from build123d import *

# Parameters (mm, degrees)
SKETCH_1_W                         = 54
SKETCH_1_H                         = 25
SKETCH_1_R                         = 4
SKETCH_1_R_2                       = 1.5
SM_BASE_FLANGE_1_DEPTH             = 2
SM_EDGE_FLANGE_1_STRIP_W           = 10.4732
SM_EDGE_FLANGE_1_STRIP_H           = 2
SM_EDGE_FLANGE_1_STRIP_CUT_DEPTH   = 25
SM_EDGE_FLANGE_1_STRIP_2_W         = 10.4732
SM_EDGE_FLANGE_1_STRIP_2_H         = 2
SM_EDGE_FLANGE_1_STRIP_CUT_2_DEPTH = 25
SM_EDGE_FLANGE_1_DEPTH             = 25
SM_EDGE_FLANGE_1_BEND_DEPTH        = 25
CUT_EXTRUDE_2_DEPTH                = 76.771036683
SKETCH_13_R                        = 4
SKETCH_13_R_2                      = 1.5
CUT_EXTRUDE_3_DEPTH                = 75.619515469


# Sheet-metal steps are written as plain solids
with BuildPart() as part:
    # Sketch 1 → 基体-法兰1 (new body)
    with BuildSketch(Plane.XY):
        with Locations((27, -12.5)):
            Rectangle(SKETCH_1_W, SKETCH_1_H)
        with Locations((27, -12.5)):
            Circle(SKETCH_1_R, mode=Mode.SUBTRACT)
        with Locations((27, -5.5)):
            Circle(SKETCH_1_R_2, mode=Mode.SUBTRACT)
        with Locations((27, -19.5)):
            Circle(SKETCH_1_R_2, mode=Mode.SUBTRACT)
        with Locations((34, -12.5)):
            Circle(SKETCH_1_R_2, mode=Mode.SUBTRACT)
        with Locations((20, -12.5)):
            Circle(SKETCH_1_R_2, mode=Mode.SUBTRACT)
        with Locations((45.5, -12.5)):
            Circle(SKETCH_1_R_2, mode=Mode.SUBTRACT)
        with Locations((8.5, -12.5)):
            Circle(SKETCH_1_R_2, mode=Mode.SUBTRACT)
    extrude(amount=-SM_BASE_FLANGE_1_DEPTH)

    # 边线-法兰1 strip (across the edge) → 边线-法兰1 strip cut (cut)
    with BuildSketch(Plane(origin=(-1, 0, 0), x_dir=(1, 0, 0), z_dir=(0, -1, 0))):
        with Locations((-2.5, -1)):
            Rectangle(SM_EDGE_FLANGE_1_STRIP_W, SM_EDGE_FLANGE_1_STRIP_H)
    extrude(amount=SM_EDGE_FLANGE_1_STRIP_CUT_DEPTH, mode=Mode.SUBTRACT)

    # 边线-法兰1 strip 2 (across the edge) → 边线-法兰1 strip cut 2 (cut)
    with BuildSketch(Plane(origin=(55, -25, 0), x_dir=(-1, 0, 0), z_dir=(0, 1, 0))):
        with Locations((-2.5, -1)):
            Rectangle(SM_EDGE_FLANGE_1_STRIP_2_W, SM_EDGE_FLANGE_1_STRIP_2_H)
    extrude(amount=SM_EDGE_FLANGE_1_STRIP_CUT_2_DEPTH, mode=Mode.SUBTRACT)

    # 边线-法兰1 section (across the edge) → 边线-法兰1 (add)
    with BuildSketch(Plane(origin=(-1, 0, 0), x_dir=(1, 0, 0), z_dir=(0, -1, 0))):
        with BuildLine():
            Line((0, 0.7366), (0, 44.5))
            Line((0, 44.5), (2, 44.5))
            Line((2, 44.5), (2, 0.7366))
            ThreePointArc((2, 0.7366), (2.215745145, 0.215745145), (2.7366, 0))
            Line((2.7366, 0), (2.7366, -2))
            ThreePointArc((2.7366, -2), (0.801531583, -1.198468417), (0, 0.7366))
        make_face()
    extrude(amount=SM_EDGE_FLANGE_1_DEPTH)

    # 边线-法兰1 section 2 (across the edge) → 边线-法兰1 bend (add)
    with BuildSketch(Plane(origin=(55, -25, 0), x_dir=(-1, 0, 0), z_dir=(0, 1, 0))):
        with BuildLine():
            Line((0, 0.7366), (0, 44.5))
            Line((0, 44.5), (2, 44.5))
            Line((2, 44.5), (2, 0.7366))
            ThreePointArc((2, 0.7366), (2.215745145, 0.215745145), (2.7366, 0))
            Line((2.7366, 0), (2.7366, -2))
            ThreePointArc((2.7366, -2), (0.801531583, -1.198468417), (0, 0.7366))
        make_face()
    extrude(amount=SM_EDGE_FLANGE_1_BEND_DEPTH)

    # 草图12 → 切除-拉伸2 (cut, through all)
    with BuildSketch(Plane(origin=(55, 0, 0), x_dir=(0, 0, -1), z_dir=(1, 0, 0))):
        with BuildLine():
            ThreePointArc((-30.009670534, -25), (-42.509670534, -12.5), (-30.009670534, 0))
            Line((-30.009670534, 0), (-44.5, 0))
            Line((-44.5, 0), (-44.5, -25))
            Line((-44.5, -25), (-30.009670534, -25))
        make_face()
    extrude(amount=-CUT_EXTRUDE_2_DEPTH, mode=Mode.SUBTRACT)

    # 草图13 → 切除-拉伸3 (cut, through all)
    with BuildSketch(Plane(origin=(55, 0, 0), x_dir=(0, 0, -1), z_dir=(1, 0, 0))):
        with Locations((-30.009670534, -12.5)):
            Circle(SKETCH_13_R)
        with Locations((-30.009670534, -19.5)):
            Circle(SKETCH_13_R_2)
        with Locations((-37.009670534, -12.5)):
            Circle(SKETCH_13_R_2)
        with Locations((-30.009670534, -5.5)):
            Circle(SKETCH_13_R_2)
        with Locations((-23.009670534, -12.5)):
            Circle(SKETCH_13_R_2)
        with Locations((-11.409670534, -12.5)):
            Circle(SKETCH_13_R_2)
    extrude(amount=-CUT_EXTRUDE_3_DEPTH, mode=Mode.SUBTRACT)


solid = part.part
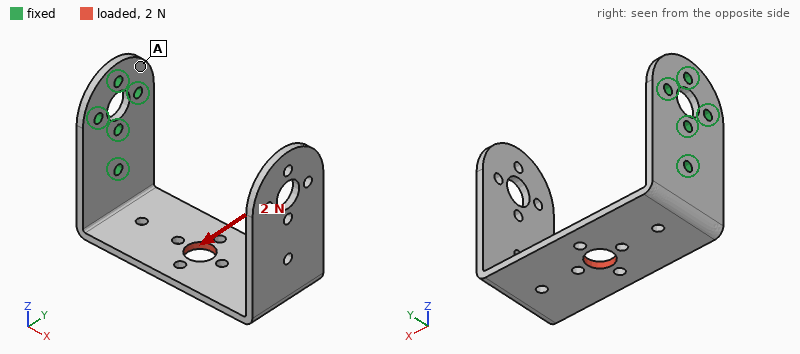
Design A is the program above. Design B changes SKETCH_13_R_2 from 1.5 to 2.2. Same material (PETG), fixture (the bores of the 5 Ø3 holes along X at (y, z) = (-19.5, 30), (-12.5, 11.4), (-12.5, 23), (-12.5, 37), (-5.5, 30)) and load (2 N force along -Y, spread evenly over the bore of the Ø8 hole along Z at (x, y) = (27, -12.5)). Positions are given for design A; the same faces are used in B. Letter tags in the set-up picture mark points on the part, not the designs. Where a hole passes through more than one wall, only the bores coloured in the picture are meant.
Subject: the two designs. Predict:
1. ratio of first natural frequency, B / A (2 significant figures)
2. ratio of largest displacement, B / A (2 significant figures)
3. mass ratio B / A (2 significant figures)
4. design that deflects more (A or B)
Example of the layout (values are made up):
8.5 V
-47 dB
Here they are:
1.0
0.88
0.97
A
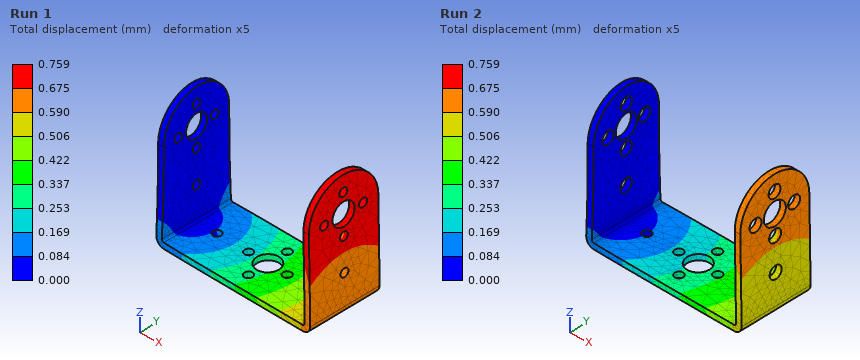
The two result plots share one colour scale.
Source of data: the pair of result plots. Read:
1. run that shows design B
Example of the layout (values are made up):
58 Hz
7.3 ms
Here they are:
Run 2
